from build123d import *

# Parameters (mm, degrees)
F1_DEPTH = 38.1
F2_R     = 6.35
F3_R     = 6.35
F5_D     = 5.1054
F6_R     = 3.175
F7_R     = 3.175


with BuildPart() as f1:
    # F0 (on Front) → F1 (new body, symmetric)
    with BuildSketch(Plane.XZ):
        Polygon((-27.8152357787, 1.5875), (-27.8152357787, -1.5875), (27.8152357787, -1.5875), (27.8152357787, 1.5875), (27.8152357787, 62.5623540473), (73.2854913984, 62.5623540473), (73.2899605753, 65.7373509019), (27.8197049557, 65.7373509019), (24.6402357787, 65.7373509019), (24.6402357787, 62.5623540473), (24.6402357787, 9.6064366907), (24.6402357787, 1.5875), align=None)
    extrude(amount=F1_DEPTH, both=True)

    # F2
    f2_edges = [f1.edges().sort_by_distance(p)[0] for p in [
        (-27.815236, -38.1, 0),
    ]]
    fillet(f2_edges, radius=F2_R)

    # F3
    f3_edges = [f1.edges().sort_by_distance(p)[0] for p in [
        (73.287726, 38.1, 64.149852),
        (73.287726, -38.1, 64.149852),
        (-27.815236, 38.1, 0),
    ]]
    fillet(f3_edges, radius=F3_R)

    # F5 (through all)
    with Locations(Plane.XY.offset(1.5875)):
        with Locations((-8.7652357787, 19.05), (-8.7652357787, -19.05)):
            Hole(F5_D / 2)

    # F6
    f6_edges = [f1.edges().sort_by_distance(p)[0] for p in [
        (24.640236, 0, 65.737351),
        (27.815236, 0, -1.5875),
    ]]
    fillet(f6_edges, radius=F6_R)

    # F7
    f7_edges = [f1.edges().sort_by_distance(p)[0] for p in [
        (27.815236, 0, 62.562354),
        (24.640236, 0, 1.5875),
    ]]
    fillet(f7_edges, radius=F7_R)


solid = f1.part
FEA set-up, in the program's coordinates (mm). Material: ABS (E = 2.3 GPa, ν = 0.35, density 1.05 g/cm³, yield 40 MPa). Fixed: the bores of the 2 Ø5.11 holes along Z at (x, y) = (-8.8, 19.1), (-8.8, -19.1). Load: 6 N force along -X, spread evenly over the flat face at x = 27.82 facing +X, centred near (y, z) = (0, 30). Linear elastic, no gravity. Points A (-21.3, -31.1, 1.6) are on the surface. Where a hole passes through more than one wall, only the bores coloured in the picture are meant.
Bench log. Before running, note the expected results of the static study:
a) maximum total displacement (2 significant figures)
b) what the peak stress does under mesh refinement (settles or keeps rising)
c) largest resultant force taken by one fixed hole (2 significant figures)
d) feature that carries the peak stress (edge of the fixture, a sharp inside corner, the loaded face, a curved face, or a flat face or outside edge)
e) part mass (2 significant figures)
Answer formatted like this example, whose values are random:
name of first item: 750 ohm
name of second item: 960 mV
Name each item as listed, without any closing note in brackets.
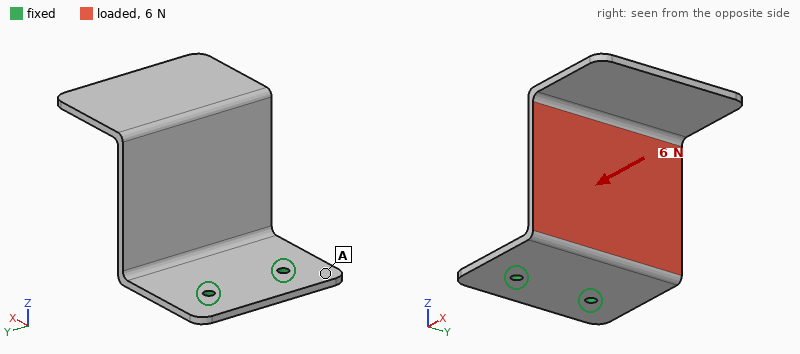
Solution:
maximum total displacement: 1.6 mm
what the peak stress does under mesh refinement: keeps rising
largest resultant force taken by one fixed hole: 3.1 N
feature that carries the peak stress: edge of the fixture
part mass: 42 g
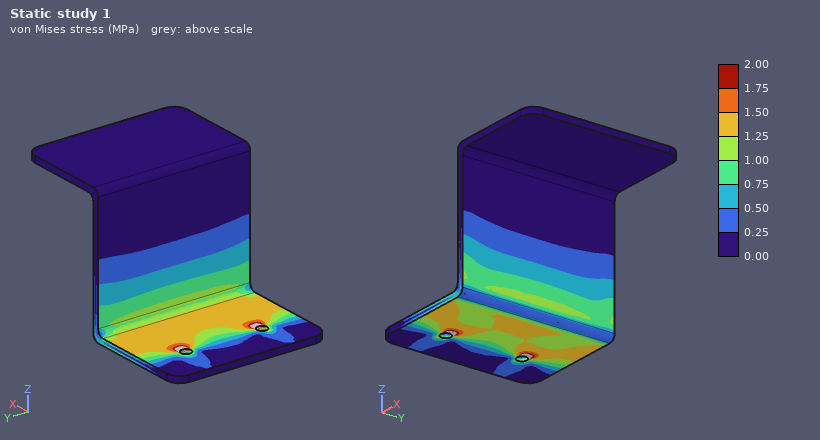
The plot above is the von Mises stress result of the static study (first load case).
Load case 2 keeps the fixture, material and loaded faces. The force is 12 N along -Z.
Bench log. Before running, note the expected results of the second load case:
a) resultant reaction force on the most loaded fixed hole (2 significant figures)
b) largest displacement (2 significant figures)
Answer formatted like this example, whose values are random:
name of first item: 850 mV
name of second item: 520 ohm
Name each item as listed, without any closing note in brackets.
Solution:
resultant reaction force on the most loaded fixed hole: 6.0 N
largest displacement: 1.7 mm
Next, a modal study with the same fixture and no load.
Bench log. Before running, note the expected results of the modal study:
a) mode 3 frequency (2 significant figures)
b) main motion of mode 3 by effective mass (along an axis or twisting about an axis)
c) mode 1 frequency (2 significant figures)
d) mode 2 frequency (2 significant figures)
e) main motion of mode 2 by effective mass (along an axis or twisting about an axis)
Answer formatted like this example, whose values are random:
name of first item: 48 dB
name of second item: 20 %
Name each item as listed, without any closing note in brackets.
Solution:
mode 3 frequency: 170 Hz
main motion of mode 3 by effective mass: twisting about Z
mode 1 frequency: 51 Hz
mode 2 frequency: 130 Hz
main motion of mode 2 by effective mass: along Y
